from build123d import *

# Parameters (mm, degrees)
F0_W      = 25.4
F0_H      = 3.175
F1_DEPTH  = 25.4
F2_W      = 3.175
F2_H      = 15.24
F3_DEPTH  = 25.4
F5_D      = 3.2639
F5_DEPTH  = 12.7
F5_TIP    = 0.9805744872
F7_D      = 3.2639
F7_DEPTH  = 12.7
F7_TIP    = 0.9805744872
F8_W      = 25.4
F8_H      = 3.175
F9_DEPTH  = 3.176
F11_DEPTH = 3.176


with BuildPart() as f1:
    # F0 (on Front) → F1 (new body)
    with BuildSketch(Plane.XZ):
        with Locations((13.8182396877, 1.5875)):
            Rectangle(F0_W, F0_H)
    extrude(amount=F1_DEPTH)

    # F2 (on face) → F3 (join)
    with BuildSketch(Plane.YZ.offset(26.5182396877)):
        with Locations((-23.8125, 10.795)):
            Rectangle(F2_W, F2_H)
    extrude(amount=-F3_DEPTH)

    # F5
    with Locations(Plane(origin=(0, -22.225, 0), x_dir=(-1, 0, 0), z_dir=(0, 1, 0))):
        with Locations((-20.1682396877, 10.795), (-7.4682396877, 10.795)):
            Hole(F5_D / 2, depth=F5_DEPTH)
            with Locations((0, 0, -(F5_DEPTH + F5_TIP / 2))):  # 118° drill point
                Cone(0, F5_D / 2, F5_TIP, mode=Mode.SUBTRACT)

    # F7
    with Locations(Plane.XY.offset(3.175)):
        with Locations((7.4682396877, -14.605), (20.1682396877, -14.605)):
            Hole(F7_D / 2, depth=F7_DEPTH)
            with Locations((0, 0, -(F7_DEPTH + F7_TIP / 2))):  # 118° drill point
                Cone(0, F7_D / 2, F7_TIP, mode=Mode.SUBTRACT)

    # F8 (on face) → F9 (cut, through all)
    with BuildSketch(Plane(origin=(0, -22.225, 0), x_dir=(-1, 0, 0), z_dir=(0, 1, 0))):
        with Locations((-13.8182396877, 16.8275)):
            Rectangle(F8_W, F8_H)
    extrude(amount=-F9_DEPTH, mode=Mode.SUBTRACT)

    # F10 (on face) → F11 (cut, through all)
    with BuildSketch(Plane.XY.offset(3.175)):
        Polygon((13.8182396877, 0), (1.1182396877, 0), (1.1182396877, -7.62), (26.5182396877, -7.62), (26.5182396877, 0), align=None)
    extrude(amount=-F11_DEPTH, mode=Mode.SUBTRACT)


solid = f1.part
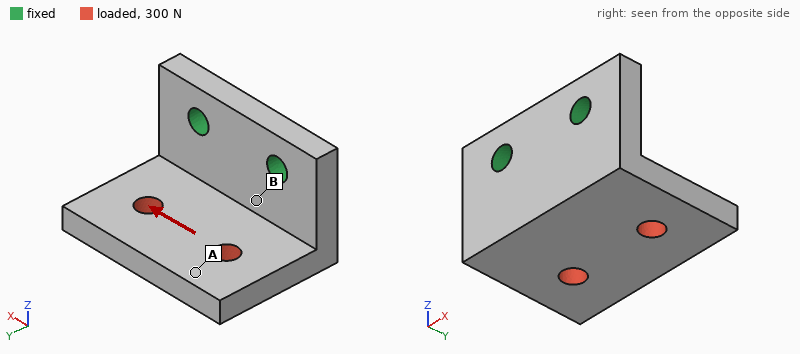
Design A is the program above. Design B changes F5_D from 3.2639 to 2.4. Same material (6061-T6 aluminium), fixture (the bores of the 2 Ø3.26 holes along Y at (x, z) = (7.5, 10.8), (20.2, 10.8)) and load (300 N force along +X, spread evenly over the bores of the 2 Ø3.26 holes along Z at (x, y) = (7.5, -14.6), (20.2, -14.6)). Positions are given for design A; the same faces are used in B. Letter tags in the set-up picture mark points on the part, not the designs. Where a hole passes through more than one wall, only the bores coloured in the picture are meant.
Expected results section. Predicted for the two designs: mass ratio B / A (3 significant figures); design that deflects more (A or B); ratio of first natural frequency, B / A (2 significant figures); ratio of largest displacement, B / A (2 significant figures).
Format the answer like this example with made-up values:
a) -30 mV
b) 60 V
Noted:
a) 1.01
b) B
c) 0.95
d) 1.1
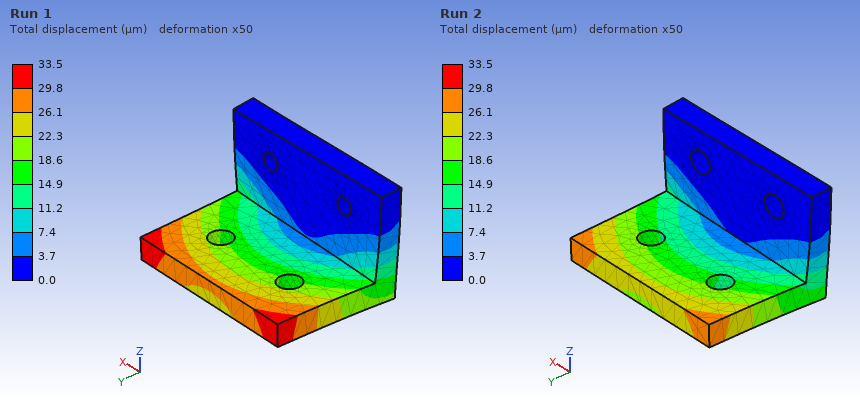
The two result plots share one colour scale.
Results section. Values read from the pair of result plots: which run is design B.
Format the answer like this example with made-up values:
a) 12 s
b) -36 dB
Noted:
a) Run 1
